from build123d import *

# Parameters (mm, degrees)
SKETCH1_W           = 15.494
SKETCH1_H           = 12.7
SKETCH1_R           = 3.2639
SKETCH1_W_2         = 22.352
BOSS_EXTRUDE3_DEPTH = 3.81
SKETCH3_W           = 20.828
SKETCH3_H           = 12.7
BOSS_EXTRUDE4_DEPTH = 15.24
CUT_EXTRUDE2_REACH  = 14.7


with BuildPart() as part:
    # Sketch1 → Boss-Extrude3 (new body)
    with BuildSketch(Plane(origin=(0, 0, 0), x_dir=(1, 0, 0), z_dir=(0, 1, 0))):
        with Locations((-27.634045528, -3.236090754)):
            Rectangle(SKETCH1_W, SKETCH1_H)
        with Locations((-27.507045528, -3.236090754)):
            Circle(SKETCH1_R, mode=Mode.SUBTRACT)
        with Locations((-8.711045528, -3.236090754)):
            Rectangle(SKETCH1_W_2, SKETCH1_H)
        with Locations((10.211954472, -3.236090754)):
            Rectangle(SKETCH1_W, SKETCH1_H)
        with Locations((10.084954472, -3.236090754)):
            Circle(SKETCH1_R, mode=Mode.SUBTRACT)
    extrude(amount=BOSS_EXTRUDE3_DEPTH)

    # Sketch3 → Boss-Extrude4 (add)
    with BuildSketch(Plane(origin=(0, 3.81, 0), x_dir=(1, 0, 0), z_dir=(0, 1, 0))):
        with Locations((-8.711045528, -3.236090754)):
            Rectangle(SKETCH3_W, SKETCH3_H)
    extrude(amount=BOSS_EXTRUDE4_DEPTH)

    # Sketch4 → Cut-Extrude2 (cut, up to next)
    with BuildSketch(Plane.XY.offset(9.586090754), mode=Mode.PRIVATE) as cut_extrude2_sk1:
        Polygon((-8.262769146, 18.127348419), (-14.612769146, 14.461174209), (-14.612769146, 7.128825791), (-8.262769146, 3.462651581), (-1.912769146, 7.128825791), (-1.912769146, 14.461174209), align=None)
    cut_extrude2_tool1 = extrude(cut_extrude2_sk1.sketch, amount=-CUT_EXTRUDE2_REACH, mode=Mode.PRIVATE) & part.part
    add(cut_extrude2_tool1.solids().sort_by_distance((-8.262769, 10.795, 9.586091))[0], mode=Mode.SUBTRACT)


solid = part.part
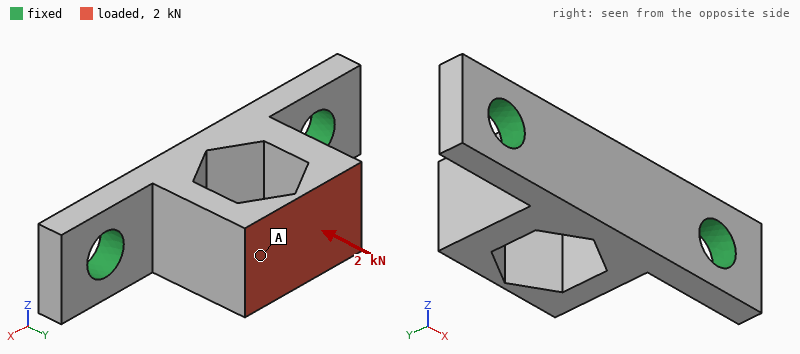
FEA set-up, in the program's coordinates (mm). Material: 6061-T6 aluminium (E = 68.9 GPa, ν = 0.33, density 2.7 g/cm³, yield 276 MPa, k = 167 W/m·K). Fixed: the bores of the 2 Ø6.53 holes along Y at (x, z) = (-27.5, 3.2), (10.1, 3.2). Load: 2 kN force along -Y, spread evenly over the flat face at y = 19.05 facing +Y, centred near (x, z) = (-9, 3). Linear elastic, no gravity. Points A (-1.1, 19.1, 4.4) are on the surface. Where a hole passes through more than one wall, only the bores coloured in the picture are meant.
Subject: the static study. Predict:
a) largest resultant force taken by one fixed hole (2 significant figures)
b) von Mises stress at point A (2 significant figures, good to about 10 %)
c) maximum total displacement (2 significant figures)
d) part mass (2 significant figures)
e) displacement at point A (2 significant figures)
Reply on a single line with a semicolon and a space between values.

1.1 kN; 20 MPa; 32 µm; 12 g; 23 µm
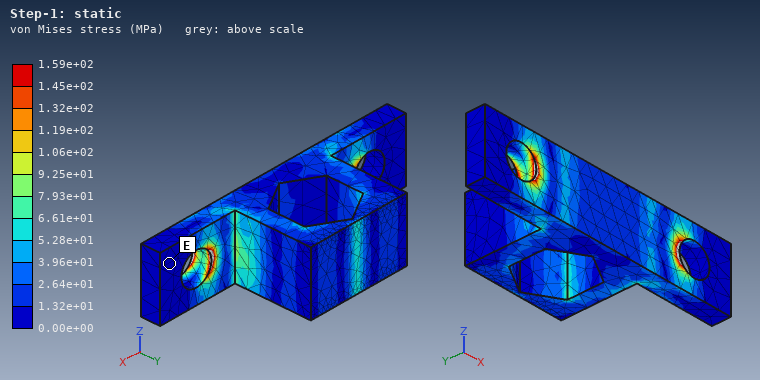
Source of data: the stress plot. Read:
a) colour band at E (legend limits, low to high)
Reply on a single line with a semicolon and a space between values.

0.00e+00 to 1.32e+01 MPa
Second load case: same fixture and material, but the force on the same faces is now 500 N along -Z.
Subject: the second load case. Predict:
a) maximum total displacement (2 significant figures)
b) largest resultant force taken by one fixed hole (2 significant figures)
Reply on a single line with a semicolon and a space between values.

90 µm; 250 N
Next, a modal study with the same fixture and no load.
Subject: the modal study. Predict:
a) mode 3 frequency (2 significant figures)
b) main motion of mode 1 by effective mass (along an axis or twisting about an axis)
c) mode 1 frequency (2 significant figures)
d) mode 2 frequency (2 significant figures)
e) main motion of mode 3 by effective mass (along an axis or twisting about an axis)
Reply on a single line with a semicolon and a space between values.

15 kHz; along Z; 7100 Hz; 14 kHz; along Y
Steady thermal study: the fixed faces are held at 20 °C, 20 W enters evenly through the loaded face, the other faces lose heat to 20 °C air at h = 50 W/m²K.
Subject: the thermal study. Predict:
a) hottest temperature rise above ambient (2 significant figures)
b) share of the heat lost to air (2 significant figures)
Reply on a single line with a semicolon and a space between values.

27 K; 7.1 %
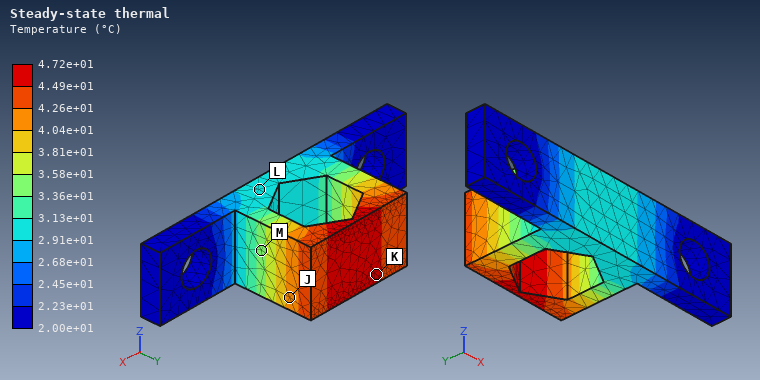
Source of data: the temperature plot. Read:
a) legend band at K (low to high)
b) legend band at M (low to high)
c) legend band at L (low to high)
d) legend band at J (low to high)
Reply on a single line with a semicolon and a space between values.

4.49e+01 to 4.72e+01 °C; 3.36e+01 to 3.58e+01 °C; 2.91e+01 to 3.13e+01 °C; 4.04e+01 to 4.26e+01 °C
